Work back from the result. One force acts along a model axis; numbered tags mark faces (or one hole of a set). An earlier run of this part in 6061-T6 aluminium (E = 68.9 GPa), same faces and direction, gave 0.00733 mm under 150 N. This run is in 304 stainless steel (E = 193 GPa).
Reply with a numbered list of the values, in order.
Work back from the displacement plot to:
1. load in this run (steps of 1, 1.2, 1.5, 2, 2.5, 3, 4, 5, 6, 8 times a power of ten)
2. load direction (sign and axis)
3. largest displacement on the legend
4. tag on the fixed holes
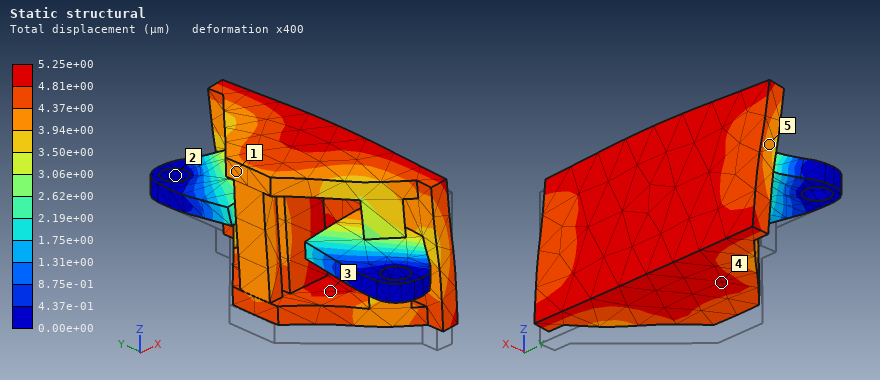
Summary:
1. 300 N
2. +Z
3. 5.25e+00 µm
4. 2
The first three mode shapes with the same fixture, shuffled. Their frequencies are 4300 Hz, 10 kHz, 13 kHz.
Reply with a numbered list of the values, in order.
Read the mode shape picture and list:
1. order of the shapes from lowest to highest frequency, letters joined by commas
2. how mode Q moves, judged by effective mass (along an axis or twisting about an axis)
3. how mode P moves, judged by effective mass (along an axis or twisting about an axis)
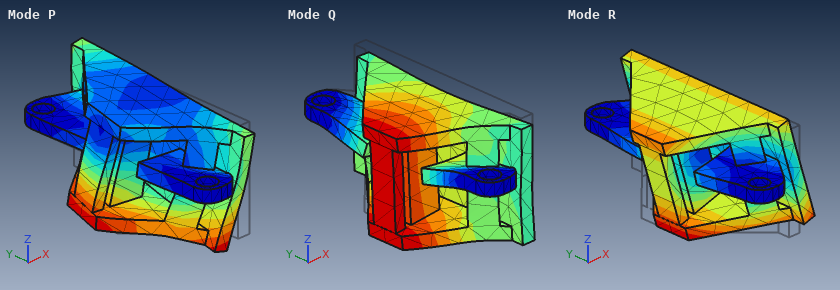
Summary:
1. R, Q, P
2. along Z
3. along Y
